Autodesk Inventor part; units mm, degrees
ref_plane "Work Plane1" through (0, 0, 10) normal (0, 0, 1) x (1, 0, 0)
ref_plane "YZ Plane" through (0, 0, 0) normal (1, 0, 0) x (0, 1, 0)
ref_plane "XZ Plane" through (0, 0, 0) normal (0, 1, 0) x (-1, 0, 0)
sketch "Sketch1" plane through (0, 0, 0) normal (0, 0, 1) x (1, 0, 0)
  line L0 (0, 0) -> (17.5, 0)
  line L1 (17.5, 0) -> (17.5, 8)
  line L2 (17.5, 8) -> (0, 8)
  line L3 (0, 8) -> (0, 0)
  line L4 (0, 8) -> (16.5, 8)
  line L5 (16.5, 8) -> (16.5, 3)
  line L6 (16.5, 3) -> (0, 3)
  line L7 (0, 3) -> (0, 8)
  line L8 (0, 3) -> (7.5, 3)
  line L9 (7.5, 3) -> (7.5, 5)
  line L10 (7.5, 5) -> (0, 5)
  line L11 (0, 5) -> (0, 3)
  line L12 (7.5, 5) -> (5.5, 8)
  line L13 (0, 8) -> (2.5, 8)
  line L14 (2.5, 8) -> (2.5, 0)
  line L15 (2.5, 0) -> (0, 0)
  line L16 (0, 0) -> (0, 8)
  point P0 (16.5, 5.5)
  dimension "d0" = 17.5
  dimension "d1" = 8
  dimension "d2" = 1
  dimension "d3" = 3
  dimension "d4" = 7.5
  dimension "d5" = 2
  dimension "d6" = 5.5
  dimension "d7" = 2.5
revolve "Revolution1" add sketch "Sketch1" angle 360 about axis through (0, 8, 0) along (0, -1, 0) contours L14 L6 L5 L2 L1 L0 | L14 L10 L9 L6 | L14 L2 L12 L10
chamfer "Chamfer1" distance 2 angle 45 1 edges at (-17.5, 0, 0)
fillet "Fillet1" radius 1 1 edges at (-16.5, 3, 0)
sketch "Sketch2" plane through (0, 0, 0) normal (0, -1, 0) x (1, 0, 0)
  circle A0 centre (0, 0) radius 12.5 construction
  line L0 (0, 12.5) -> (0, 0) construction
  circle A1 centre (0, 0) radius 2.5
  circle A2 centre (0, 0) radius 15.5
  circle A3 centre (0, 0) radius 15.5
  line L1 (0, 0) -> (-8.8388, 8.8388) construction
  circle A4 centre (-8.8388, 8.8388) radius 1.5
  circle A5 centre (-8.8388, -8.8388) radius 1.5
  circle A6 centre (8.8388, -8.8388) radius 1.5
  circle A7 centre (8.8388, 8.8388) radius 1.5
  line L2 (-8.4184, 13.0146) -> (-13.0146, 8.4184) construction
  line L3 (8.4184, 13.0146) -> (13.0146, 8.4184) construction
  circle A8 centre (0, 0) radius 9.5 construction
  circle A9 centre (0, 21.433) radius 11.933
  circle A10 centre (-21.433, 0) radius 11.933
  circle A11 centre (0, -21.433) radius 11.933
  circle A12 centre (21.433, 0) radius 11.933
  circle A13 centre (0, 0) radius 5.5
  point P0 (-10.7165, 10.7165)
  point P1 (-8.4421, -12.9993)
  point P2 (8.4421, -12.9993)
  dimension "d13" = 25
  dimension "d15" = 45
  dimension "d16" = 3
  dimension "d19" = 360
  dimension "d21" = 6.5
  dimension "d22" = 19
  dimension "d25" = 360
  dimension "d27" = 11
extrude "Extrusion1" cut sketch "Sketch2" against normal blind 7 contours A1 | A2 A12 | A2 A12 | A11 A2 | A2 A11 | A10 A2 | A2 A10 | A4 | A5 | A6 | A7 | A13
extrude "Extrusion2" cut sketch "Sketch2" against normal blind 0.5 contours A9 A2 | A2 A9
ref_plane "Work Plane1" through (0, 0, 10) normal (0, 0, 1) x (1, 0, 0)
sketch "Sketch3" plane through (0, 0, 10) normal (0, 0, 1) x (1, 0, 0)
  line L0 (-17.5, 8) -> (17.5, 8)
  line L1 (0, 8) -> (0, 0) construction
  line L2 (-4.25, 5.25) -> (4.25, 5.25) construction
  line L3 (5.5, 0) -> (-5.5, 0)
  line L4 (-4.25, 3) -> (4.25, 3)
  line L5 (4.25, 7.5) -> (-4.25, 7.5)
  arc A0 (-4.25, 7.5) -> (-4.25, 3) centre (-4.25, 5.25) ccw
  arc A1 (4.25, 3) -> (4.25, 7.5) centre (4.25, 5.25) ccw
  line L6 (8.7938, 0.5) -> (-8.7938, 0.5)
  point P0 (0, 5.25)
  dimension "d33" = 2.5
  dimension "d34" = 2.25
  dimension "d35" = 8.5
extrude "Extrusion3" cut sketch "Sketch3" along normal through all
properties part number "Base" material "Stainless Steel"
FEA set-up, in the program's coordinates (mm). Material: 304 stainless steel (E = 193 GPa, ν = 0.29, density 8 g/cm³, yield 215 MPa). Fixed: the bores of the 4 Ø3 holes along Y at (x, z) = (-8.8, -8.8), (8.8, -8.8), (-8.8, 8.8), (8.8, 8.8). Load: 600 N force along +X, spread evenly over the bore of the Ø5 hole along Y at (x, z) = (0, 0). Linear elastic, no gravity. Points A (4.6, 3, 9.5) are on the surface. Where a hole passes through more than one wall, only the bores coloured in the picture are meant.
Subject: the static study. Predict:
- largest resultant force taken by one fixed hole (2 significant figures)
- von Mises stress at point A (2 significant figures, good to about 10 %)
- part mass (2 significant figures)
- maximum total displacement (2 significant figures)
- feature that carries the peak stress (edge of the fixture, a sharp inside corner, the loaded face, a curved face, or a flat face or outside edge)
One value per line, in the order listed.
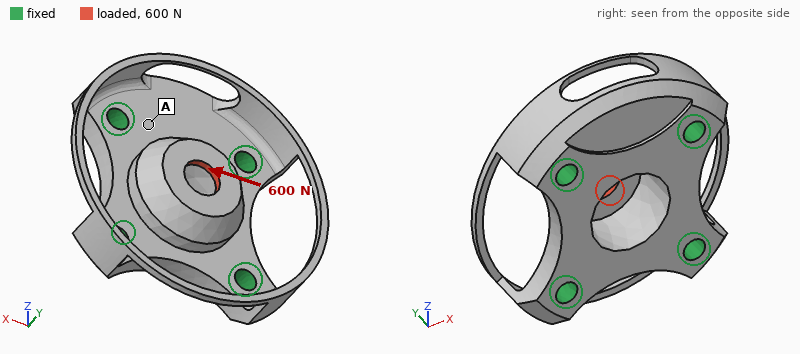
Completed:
210 N
10 MPa
16 g
4.4 µm
the loaded face
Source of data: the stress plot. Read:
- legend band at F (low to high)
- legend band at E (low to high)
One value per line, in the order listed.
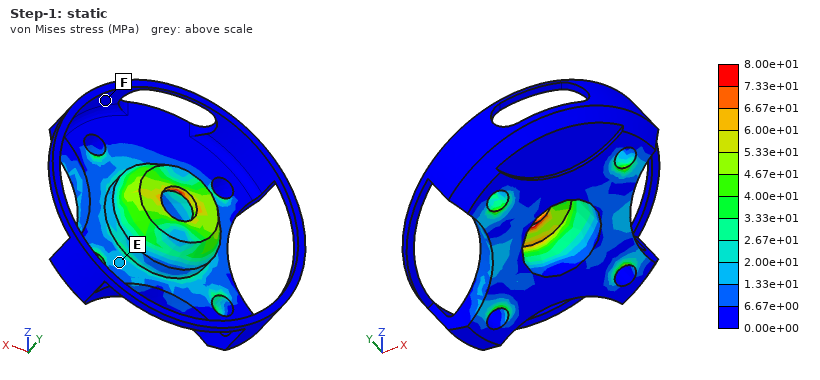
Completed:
0.00e+00 to 6.67e+00 MPa
1.33e+01 to 2.00e+01 MPa
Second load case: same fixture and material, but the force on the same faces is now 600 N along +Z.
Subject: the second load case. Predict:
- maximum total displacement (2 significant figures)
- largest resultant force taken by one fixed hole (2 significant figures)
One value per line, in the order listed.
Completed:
4.3 µm
200 N
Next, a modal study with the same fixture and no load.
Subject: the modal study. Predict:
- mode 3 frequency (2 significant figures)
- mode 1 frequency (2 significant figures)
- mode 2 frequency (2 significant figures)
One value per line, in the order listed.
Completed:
10 kHz
10 kHz
10 kHz
